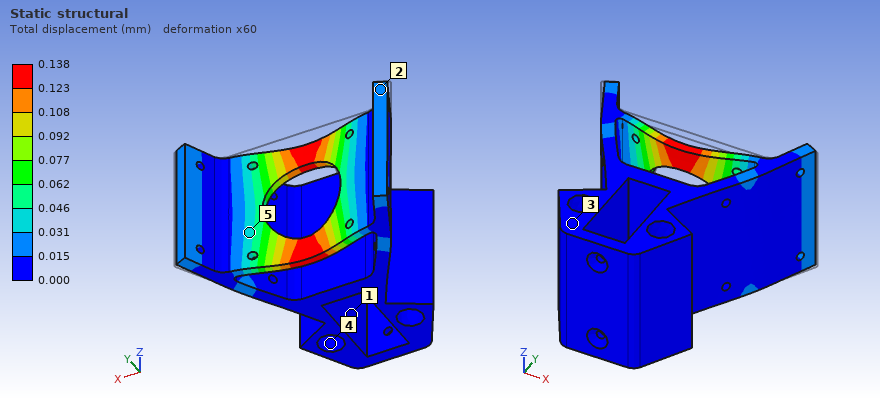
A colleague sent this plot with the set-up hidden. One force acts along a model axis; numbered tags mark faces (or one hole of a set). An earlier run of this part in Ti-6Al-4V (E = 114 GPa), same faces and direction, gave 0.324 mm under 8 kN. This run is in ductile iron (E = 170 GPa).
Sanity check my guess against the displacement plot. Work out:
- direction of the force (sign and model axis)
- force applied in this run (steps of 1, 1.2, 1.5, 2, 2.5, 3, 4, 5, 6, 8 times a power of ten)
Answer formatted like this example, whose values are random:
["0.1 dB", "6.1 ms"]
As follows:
["-Y", "5 kN"]
